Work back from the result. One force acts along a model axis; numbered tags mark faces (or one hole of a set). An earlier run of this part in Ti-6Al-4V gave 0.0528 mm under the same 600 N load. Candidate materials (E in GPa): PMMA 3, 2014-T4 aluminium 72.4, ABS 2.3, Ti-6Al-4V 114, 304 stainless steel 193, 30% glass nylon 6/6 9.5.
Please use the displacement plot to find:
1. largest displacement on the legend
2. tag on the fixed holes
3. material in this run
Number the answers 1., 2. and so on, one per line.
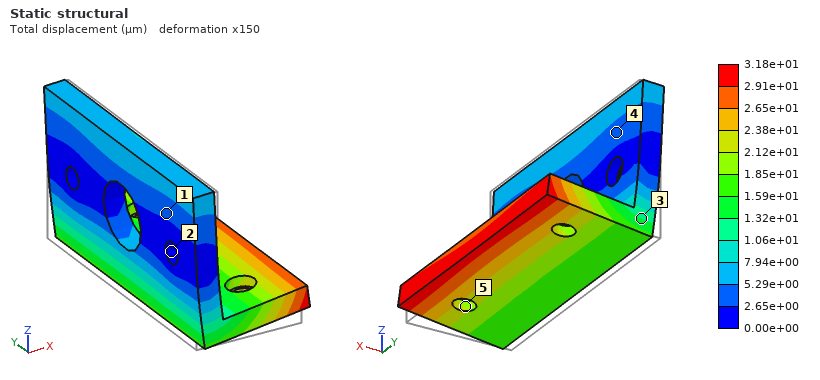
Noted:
1. 3.18e+01 µm
2. 2
3. 304 stainless steel
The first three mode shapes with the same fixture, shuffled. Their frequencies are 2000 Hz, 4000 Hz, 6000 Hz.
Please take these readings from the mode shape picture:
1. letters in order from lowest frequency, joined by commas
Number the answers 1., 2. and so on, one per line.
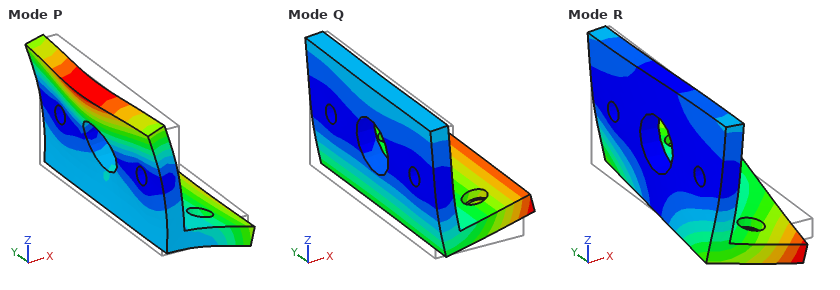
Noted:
1. Q, R, P
